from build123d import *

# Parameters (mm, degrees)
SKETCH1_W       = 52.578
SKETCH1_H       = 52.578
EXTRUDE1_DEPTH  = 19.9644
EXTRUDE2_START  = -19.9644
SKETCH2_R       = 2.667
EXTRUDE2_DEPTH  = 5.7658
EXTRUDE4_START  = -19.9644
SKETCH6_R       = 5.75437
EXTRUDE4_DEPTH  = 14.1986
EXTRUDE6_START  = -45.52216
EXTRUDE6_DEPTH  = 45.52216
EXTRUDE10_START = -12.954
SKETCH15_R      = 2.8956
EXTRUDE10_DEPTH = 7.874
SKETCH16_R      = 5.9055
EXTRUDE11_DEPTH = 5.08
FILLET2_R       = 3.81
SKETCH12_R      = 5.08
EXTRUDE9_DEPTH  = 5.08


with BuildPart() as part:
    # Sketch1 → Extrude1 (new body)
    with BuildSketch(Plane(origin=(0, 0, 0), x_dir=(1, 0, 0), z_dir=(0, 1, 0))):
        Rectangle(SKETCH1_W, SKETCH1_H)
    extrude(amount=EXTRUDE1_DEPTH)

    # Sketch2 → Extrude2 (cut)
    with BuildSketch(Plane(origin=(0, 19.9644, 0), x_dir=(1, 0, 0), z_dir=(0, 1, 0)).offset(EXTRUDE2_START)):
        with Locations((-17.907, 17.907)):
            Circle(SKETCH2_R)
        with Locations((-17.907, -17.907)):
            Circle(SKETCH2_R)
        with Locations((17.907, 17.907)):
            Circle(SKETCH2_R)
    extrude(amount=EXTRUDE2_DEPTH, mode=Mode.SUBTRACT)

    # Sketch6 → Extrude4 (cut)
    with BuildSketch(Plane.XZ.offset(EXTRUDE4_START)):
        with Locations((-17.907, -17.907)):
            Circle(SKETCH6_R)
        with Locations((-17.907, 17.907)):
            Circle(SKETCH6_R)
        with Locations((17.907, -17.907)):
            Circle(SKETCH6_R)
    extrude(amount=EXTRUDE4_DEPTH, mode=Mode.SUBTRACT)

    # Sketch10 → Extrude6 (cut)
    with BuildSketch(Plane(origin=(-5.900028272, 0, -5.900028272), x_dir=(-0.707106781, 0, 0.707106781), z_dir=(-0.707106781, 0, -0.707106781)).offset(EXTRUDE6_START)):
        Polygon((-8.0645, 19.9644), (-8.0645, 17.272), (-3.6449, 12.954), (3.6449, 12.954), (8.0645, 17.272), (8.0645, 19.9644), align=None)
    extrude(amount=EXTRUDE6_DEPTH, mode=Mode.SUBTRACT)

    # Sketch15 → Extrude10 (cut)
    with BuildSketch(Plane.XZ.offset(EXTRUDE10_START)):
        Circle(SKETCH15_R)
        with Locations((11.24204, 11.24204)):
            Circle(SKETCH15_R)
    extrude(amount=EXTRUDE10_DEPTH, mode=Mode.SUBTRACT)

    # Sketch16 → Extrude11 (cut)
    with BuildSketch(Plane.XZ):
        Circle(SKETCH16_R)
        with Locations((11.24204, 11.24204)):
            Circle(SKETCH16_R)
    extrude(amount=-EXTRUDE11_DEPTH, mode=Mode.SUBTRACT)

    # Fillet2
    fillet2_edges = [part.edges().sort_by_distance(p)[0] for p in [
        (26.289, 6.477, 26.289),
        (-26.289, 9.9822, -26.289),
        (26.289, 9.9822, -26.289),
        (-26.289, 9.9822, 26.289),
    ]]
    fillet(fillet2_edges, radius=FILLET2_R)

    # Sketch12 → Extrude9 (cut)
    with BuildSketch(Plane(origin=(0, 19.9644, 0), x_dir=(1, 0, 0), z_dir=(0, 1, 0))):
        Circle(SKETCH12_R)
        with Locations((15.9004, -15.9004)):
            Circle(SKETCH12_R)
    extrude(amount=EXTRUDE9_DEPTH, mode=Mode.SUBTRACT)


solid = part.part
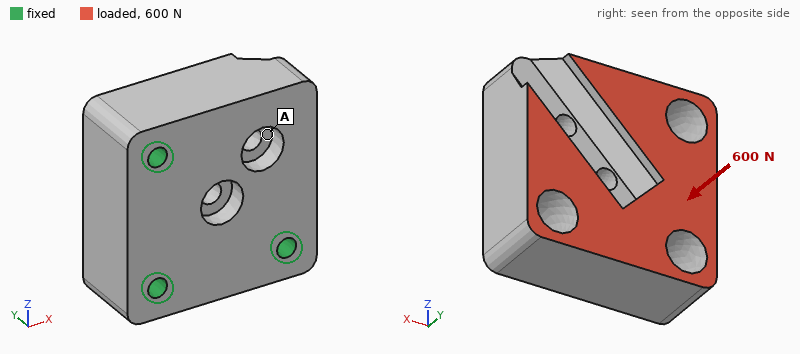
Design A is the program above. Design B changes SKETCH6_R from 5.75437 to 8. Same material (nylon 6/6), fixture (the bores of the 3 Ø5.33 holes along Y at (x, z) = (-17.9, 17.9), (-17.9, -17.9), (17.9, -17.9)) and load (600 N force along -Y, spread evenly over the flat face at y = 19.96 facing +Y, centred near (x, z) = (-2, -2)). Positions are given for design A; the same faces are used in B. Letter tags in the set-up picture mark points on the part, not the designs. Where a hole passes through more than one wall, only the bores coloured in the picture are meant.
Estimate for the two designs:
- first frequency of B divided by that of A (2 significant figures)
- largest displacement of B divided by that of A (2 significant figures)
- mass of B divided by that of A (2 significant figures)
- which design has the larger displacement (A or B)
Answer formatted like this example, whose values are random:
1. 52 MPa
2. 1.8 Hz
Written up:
1. 0.92
2. 1.4
3. 0.91
4. B
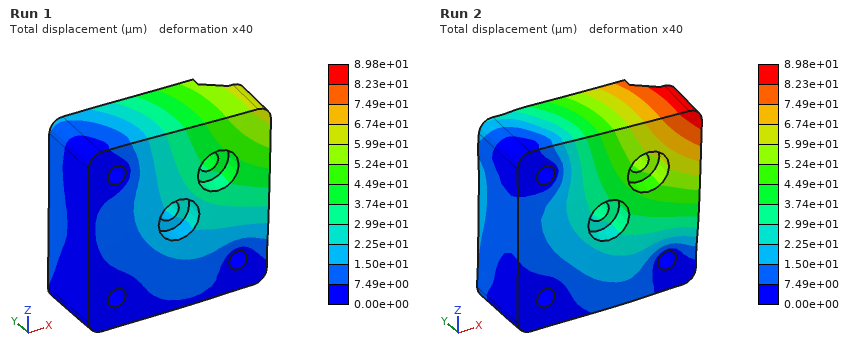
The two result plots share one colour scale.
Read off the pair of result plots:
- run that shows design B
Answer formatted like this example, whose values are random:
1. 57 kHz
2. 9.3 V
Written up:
1. Run 2
